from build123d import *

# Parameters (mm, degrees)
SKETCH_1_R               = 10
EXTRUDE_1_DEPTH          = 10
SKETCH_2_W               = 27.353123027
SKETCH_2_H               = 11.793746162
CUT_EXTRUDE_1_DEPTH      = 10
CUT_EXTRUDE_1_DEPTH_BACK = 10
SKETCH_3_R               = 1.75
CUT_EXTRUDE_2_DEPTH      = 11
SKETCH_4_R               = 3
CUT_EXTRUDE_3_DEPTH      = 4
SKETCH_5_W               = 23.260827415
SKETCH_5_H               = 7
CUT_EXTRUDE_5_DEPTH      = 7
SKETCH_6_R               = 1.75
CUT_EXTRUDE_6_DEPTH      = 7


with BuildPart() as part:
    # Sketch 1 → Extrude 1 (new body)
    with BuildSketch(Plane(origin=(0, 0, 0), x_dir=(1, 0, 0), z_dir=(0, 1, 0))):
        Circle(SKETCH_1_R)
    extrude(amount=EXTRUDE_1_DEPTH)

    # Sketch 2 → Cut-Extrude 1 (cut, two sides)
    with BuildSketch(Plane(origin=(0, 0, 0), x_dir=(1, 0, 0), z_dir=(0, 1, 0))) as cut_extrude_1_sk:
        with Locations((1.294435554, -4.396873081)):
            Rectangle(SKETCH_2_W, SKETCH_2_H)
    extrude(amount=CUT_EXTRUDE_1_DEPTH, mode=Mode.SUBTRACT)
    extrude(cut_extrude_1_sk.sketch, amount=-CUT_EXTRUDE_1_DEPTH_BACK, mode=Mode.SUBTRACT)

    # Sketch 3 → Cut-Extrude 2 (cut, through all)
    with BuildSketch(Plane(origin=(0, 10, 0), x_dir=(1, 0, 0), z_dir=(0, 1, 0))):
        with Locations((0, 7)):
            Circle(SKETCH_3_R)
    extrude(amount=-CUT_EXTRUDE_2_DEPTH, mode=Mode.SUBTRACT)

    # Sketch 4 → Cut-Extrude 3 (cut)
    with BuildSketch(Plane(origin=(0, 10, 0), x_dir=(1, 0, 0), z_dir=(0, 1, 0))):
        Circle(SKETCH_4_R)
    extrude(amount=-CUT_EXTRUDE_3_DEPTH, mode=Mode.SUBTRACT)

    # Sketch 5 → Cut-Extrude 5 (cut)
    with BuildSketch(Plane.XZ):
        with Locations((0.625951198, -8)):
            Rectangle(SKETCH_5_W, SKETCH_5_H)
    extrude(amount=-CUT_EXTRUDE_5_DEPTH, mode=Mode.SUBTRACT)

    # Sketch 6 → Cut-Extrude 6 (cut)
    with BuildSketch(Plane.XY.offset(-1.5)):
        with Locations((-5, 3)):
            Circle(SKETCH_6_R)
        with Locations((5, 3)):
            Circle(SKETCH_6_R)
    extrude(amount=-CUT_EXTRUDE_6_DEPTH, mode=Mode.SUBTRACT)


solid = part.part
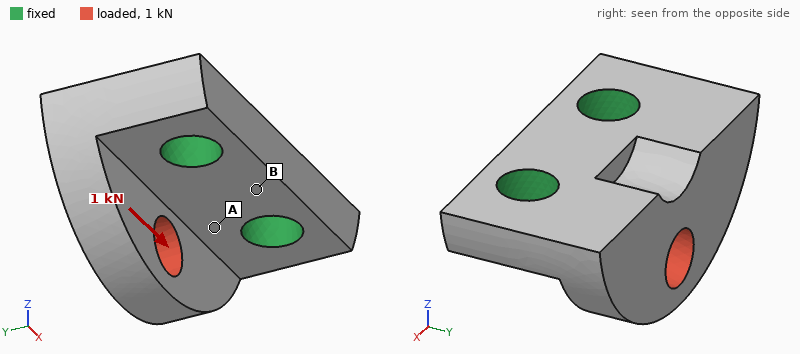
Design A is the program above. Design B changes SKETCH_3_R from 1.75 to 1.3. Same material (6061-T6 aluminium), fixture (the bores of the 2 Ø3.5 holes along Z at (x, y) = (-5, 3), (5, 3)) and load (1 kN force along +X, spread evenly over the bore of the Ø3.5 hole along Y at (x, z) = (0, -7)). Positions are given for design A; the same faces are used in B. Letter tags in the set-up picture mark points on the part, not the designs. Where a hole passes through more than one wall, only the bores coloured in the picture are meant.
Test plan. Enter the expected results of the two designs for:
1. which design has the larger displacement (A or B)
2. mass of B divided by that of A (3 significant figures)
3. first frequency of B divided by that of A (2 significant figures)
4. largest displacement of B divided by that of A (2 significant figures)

A
1.02
0.98
0.89
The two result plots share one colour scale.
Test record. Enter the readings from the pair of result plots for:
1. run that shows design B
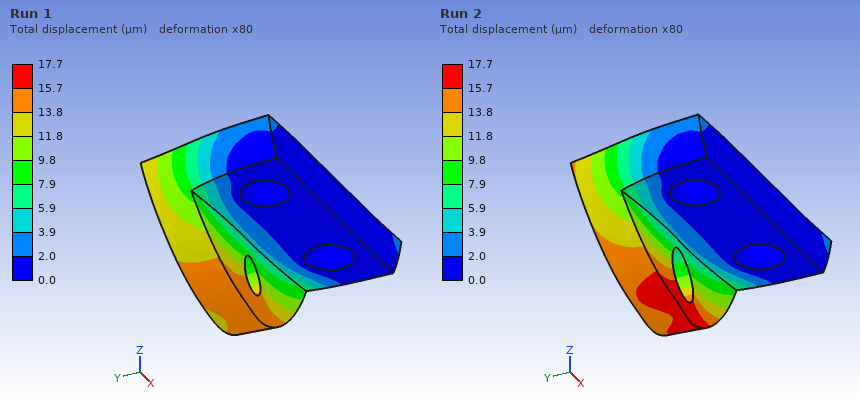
Run 1
